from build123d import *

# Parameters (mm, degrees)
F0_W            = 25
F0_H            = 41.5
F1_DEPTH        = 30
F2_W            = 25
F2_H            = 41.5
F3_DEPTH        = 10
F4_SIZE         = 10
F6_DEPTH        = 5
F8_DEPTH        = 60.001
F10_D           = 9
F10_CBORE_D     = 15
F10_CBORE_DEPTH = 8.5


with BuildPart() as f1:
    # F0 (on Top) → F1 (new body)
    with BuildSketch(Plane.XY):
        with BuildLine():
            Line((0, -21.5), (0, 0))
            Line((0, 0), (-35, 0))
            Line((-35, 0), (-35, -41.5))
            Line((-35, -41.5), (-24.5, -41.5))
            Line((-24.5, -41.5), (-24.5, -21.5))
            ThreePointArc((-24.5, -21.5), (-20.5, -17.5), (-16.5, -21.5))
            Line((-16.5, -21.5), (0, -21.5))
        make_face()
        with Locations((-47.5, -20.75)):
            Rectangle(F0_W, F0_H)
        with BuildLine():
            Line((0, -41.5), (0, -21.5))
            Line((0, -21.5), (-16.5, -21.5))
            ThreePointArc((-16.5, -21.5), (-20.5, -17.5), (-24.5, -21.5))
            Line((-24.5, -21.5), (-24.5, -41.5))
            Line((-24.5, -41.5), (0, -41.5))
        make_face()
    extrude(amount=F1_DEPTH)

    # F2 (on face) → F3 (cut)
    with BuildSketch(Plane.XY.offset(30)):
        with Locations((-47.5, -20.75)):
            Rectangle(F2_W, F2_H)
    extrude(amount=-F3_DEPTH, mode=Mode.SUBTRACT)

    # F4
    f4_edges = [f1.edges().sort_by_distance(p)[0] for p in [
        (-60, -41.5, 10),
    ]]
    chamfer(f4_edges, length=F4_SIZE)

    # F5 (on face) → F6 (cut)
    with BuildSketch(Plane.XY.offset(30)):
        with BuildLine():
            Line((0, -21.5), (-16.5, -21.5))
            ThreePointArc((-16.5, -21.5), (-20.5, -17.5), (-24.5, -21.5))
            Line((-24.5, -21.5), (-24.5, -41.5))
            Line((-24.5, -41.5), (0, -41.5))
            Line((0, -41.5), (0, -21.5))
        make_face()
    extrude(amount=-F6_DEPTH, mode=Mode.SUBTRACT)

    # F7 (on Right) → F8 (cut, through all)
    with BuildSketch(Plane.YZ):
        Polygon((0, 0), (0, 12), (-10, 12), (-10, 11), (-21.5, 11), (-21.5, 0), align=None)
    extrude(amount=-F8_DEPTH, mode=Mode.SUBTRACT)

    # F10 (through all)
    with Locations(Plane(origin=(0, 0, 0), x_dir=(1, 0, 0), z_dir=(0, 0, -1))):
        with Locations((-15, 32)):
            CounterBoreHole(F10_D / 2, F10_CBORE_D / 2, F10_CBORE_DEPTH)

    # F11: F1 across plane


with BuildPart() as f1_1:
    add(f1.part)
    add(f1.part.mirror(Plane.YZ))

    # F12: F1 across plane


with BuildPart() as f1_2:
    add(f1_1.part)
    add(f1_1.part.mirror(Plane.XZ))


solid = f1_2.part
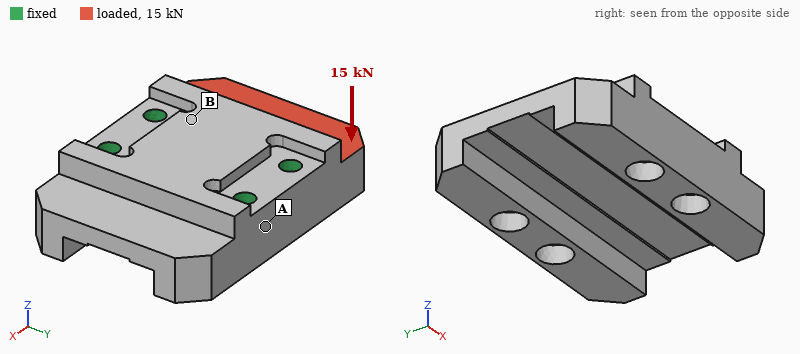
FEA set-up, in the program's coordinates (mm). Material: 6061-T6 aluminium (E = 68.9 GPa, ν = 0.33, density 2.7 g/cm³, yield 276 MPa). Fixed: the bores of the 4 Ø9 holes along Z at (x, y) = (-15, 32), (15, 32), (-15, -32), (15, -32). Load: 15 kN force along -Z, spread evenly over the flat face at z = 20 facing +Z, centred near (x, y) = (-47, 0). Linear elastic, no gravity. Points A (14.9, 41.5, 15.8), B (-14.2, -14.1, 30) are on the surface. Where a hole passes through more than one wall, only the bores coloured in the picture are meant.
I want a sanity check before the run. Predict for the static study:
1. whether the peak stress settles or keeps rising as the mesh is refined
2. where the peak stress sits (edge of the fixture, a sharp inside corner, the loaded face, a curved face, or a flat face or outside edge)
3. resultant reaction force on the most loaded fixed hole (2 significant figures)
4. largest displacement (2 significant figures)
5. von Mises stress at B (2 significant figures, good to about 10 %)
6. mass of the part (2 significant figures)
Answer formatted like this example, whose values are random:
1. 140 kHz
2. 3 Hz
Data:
1. keeps rising
2. edge of the fixture
3. 10 kN
4. 0.18 mm
5. 48 MPa
6. 470 g
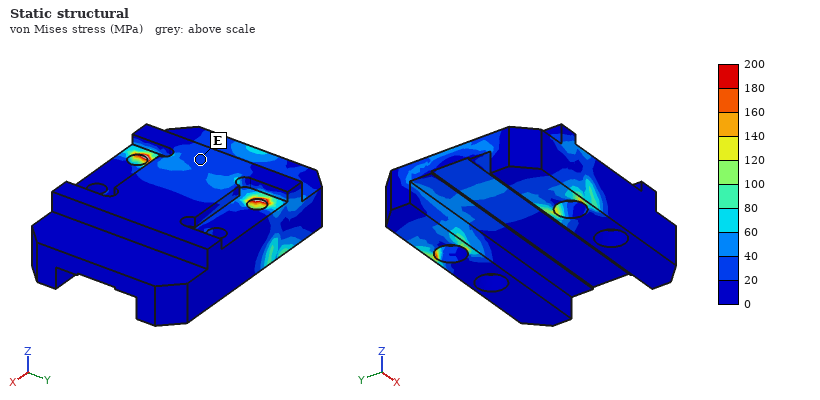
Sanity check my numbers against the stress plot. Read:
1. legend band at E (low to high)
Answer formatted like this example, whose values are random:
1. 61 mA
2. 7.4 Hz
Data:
1. 20 to 40 MPa
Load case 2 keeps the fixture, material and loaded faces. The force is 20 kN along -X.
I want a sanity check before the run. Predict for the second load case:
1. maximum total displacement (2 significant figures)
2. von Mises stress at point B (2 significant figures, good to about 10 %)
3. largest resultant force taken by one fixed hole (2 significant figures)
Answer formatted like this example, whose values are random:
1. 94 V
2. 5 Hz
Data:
1. 58 µm
2. 9.1 MPa
3. 7.8 kN
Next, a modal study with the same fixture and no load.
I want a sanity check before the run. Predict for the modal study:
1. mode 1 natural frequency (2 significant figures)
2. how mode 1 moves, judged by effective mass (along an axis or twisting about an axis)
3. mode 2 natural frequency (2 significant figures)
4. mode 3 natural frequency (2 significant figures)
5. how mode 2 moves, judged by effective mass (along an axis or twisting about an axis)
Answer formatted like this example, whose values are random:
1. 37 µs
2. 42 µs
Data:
1. 6700 Hz
2. twisting about Y
3. 7200 Hz
4. 8800 Hz
5. along Z
